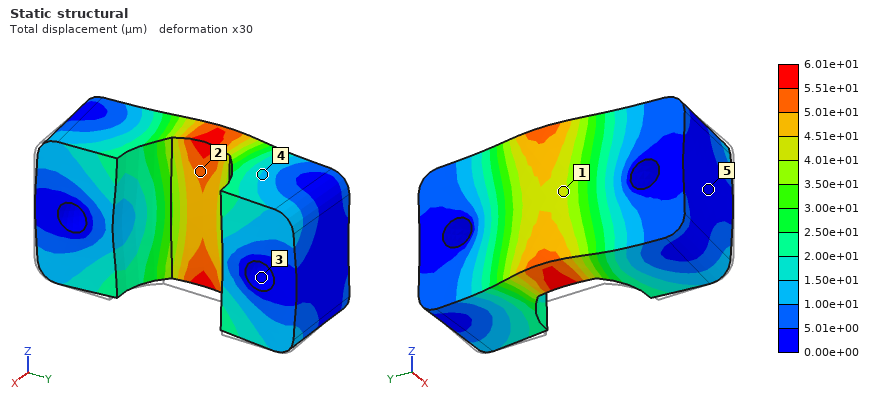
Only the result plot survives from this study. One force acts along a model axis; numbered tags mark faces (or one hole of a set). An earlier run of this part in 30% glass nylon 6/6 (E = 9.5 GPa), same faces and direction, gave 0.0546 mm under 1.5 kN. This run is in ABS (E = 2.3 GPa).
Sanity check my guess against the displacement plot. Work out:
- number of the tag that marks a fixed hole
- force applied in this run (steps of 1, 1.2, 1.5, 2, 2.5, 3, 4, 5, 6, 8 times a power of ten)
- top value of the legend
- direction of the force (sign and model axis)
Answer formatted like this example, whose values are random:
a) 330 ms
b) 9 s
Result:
a) 3
b) 400 N
c) 6.01e+01 µm
d) -X
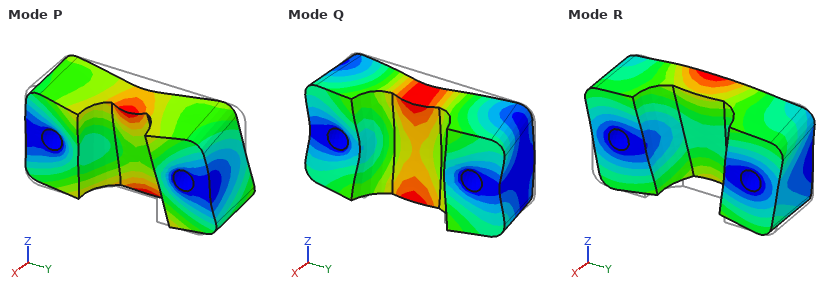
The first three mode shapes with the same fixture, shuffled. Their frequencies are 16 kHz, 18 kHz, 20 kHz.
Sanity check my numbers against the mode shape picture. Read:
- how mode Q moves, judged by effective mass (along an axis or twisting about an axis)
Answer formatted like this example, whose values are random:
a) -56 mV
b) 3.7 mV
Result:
a) along X
